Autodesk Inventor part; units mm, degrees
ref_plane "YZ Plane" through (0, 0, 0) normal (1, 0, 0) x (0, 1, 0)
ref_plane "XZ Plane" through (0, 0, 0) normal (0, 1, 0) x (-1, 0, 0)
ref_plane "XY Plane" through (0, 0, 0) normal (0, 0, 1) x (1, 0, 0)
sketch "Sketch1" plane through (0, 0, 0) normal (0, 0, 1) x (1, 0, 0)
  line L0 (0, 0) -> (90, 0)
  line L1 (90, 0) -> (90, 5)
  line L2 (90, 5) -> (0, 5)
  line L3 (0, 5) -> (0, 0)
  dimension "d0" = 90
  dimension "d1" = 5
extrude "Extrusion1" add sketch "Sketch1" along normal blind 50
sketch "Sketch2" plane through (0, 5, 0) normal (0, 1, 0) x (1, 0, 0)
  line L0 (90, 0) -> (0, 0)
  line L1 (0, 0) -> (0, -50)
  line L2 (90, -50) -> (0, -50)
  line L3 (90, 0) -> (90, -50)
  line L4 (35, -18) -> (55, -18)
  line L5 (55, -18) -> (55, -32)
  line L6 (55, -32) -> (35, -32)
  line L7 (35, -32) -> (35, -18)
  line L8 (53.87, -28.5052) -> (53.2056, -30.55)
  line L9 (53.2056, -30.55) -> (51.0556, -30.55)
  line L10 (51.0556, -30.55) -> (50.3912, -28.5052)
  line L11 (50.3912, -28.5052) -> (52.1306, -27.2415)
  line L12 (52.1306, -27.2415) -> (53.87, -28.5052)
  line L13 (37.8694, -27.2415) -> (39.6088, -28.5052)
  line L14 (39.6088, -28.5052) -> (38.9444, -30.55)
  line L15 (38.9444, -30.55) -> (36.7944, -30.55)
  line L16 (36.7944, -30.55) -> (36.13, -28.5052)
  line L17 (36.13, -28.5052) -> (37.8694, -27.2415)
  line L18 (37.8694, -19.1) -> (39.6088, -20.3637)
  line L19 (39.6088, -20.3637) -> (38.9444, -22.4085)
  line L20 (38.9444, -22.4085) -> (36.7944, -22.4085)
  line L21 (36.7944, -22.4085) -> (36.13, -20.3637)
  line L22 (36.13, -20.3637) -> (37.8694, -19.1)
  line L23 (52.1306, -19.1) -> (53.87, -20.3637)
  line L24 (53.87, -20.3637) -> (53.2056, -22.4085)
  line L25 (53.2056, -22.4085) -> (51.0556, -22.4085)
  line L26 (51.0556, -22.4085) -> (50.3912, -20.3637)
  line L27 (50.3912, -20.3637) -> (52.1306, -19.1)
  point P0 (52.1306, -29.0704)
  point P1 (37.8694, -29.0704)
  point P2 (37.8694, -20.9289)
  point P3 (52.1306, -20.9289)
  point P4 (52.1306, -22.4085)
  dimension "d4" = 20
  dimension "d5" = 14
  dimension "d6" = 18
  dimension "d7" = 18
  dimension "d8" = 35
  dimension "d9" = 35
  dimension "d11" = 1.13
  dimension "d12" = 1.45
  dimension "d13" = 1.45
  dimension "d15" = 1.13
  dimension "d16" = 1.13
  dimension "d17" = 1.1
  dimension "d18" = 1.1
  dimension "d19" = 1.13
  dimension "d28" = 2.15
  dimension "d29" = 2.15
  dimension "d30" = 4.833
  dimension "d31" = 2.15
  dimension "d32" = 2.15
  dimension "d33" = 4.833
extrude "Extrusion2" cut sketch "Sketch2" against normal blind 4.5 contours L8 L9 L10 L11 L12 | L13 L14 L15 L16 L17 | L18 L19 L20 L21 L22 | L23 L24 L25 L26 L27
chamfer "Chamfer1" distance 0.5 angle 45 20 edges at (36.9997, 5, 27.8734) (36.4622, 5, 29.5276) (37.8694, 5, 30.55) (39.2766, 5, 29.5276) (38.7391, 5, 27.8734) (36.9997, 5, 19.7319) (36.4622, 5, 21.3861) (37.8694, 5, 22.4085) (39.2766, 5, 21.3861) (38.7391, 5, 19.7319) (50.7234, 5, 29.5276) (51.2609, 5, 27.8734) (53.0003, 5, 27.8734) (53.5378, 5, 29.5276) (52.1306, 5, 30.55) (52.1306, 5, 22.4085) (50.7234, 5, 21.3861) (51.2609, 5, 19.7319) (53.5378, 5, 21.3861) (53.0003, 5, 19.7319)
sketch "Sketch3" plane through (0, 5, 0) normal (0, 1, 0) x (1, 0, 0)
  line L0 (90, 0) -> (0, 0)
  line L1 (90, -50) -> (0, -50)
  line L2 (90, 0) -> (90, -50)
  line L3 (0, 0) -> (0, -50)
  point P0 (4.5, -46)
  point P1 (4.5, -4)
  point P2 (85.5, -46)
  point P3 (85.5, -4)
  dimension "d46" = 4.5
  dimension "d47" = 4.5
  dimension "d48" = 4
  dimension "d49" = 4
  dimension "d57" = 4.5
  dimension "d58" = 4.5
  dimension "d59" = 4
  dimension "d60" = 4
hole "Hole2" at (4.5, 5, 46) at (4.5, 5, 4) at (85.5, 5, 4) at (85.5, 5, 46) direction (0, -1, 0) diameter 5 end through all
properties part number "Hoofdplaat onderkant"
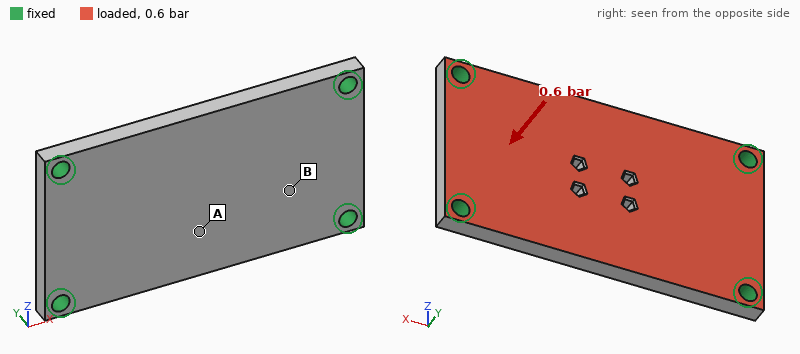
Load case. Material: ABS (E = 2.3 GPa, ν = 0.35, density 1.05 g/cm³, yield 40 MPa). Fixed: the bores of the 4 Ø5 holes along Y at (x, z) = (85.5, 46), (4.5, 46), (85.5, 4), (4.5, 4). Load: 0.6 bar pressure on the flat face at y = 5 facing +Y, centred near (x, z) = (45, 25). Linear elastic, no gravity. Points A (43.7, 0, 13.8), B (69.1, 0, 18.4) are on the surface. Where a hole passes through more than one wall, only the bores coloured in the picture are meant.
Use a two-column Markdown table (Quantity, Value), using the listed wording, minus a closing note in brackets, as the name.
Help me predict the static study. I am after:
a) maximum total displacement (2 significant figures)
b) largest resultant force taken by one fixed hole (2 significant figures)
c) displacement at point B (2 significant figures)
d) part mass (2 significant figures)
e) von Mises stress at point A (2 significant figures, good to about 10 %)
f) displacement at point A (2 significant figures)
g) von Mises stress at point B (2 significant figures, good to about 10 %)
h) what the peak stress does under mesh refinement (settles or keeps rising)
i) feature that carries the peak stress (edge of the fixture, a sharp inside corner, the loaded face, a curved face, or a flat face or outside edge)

| Quantity | Value |
|---|---|
| maximum total displacement | 0.36 mm |
| largest resultant force taken by one fixed hole | 65 N |
| displacement at point B | 0.18 mm |
| part mass | 23 g |
| von Mises stress at point A | 3.9 MPa |
| displacement at point A | 0.35 mm |
| von Mises stress at point B | 1.3 MPa |
| what the peak stress does under mesh refinement | keeps rising |
| feature that carries the peak stress | edge of the fixture |
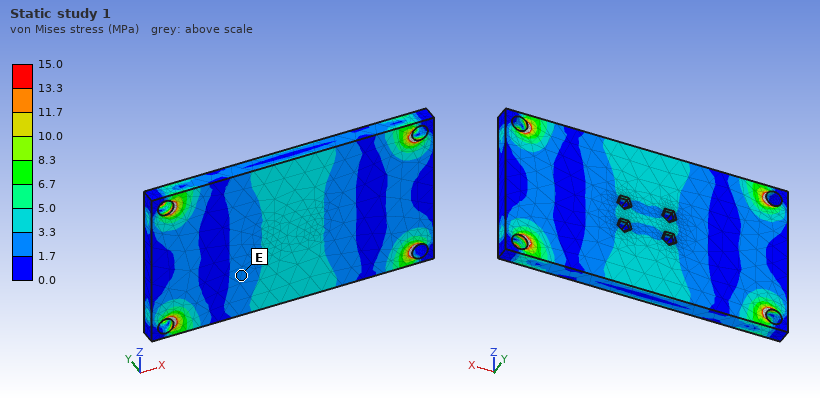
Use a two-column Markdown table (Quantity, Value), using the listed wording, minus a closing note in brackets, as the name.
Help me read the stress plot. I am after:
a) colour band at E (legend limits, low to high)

| Quantity | Value |
|---|---|
| colour band at E | 1.7 to 3.3 MPa |
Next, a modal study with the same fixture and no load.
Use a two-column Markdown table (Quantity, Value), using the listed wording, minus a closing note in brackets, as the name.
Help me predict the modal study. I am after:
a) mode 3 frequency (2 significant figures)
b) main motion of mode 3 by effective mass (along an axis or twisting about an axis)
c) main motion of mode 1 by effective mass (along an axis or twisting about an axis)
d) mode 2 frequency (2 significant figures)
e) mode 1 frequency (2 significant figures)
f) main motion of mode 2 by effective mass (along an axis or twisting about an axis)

| Quantity | Value |
|---|---|
| mode 3 frequency | 2700 Hz |
| main motion of mode 3 by effective mass | twisting about Z |
| main motion of mode 1 by effective mass | along Y |
| mode 2 frequency | 1700 Hz |
| mode 1 frequency | 1000 Hz |
| main motion of mode 2 by effective mass | twisting about X |
